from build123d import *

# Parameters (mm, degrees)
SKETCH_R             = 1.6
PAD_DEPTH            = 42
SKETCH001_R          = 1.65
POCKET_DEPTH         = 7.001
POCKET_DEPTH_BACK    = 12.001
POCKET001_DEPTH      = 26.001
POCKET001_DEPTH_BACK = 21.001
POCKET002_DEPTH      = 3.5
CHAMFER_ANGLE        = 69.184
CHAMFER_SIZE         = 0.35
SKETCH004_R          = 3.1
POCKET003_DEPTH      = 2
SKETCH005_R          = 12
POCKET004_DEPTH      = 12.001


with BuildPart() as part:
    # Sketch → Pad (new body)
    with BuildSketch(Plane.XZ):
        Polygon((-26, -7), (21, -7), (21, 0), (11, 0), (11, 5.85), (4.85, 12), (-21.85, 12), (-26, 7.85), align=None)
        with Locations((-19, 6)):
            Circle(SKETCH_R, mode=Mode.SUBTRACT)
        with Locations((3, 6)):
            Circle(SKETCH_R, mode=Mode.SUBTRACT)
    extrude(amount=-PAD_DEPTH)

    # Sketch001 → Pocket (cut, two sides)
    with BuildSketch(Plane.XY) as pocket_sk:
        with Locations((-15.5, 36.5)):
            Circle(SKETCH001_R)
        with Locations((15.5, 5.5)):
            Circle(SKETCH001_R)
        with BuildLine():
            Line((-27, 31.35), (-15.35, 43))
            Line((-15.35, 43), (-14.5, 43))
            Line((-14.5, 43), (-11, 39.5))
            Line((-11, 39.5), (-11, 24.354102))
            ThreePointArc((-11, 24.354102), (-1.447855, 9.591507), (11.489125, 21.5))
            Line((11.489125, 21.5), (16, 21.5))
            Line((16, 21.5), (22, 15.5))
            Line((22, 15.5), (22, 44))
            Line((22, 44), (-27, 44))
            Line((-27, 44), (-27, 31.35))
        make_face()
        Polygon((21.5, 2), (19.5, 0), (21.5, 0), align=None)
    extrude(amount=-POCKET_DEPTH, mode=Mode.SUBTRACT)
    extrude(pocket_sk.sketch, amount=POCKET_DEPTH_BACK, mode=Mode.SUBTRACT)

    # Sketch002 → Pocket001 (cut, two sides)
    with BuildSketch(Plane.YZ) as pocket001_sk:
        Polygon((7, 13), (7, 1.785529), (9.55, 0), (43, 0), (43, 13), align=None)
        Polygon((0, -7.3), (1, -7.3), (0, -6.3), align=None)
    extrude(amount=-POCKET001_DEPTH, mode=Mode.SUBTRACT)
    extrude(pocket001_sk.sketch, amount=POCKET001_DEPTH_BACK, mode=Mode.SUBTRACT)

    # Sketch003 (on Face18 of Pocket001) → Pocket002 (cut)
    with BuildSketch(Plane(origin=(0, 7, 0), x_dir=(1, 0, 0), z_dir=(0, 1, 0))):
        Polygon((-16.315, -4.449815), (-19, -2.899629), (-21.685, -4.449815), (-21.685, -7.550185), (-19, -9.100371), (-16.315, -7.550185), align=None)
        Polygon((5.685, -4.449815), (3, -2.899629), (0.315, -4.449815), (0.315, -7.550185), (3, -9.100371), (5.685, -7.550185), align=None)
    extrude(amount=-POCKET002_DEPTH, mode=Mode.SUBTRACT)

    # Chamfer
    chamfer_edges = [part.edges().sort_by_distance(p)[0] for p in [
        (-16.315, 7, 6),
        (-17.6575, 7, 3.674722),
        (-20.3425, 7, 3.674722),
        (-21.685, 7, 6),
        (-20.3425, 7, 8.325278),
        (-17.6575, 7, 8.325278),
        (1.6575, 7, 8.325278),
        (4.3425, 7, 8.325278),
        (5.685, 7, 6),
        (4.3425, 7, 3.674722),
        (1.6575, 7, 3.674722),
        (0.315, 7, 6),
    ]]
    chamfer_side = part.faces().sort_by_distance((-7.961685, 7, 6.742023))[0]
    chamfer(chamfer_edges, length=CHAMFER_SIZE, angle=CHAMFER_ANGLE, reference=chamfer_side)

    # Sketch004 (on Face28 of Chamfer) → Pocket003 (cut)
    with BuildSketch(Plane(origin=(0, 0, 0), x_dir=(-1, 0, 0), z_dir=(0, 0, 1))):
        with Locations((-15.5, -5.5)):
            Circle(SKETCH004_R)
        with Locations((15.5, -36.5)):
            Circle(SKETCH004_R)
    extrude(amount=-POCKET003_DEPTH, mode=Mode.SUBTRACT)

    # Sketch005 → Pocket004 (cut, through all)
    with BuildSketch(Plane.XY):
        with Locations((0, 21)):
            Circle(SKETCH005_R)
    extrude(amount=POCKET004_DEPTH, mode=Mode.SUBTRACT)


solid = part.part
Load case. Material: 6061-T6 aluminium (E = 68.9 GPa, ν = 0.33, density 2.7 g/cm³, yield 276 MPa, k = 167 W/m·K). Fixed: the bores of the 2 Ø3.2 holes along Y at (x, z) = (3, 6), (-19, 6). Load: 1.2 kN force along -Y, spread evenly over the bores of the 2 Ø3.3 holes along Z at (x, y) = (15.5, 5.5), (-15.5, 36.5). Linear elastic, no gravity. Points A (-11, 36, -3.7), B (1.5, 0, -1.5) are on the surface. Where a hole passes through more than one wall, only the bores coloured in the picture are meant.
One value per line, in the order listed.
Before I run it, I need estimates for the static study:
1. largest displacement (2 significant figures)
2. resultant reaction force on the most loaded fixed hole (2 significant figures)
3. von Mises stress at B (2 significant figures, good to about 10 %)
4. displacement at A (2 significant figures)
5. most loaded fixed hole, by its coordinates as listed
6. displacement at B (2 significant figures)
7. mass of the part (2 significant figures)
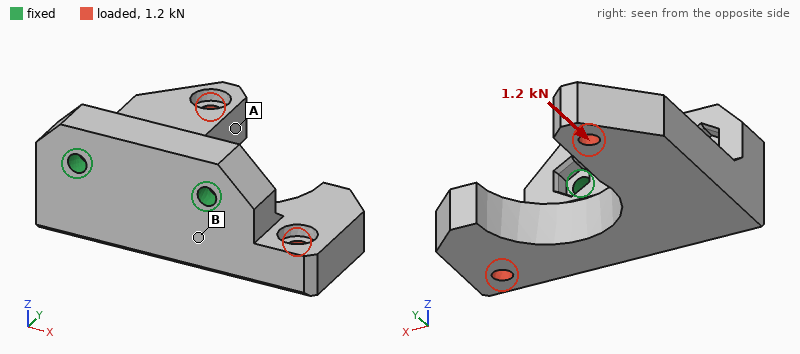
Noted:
0.14 mm
980 N
38 MPa
0.11 mm
(3, 6)
0.026 mm
26 g
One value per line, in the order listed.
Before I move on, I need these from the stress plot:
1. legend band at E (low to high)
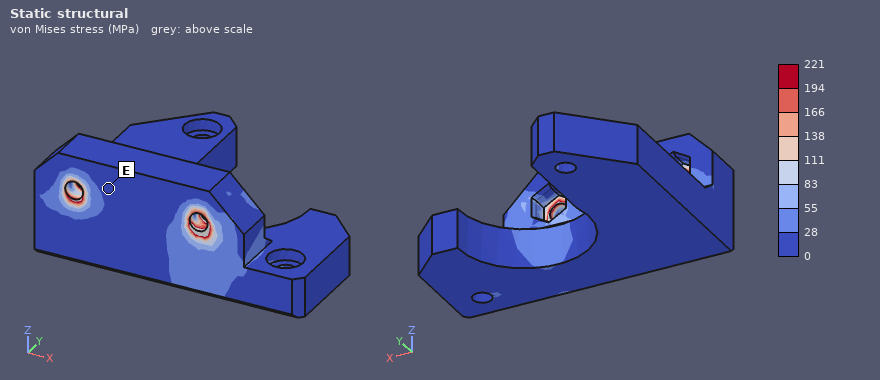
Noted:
0 to 28 MPa
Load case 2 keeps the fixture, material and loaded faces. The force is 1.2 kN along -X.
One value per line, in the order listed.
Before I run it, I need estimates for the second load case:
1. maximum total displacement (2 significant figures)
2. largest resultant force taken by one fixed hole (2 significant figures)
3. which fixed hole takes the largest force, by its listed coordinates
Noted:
0.10 mm
1.4 kN
(3, 6)
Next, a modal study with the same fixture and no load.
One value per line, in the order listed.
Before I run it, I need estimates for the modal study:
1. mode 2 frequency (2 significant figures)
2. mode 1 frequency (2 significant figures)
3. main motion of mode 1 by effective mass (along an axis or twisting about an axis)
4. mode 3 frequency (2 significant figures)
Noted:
6500 Hz
3100 Hz
along Z
8400 Hz
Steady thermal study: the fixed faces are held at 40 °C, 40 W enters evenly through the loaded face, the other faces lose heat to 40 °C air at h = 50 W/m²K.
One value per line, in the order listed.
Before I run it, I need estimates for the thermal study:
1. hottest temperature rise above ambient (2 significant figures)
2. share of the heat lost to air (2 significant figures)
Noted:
49 K
9.5 %
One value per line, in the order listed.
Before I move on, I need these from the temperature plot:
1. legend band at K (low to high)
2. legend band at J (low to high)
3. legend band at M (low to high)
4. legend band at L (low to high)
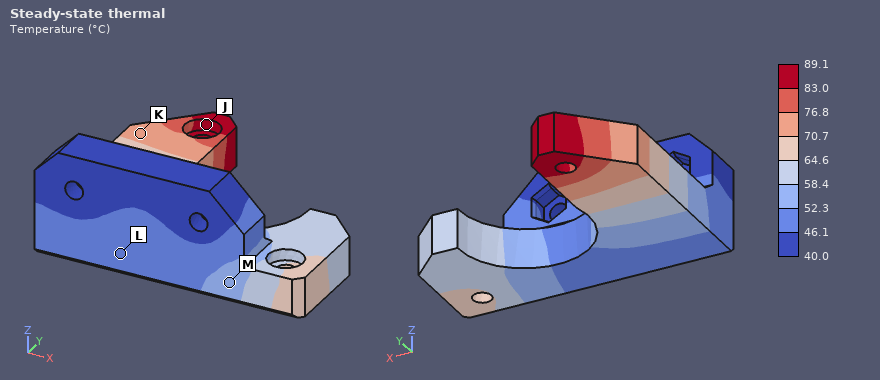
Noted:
70.7 to 76.8 °C
83.0 to 89.1 °C
52.3 to 58.4 °C
46.1 to 52.3 °C
